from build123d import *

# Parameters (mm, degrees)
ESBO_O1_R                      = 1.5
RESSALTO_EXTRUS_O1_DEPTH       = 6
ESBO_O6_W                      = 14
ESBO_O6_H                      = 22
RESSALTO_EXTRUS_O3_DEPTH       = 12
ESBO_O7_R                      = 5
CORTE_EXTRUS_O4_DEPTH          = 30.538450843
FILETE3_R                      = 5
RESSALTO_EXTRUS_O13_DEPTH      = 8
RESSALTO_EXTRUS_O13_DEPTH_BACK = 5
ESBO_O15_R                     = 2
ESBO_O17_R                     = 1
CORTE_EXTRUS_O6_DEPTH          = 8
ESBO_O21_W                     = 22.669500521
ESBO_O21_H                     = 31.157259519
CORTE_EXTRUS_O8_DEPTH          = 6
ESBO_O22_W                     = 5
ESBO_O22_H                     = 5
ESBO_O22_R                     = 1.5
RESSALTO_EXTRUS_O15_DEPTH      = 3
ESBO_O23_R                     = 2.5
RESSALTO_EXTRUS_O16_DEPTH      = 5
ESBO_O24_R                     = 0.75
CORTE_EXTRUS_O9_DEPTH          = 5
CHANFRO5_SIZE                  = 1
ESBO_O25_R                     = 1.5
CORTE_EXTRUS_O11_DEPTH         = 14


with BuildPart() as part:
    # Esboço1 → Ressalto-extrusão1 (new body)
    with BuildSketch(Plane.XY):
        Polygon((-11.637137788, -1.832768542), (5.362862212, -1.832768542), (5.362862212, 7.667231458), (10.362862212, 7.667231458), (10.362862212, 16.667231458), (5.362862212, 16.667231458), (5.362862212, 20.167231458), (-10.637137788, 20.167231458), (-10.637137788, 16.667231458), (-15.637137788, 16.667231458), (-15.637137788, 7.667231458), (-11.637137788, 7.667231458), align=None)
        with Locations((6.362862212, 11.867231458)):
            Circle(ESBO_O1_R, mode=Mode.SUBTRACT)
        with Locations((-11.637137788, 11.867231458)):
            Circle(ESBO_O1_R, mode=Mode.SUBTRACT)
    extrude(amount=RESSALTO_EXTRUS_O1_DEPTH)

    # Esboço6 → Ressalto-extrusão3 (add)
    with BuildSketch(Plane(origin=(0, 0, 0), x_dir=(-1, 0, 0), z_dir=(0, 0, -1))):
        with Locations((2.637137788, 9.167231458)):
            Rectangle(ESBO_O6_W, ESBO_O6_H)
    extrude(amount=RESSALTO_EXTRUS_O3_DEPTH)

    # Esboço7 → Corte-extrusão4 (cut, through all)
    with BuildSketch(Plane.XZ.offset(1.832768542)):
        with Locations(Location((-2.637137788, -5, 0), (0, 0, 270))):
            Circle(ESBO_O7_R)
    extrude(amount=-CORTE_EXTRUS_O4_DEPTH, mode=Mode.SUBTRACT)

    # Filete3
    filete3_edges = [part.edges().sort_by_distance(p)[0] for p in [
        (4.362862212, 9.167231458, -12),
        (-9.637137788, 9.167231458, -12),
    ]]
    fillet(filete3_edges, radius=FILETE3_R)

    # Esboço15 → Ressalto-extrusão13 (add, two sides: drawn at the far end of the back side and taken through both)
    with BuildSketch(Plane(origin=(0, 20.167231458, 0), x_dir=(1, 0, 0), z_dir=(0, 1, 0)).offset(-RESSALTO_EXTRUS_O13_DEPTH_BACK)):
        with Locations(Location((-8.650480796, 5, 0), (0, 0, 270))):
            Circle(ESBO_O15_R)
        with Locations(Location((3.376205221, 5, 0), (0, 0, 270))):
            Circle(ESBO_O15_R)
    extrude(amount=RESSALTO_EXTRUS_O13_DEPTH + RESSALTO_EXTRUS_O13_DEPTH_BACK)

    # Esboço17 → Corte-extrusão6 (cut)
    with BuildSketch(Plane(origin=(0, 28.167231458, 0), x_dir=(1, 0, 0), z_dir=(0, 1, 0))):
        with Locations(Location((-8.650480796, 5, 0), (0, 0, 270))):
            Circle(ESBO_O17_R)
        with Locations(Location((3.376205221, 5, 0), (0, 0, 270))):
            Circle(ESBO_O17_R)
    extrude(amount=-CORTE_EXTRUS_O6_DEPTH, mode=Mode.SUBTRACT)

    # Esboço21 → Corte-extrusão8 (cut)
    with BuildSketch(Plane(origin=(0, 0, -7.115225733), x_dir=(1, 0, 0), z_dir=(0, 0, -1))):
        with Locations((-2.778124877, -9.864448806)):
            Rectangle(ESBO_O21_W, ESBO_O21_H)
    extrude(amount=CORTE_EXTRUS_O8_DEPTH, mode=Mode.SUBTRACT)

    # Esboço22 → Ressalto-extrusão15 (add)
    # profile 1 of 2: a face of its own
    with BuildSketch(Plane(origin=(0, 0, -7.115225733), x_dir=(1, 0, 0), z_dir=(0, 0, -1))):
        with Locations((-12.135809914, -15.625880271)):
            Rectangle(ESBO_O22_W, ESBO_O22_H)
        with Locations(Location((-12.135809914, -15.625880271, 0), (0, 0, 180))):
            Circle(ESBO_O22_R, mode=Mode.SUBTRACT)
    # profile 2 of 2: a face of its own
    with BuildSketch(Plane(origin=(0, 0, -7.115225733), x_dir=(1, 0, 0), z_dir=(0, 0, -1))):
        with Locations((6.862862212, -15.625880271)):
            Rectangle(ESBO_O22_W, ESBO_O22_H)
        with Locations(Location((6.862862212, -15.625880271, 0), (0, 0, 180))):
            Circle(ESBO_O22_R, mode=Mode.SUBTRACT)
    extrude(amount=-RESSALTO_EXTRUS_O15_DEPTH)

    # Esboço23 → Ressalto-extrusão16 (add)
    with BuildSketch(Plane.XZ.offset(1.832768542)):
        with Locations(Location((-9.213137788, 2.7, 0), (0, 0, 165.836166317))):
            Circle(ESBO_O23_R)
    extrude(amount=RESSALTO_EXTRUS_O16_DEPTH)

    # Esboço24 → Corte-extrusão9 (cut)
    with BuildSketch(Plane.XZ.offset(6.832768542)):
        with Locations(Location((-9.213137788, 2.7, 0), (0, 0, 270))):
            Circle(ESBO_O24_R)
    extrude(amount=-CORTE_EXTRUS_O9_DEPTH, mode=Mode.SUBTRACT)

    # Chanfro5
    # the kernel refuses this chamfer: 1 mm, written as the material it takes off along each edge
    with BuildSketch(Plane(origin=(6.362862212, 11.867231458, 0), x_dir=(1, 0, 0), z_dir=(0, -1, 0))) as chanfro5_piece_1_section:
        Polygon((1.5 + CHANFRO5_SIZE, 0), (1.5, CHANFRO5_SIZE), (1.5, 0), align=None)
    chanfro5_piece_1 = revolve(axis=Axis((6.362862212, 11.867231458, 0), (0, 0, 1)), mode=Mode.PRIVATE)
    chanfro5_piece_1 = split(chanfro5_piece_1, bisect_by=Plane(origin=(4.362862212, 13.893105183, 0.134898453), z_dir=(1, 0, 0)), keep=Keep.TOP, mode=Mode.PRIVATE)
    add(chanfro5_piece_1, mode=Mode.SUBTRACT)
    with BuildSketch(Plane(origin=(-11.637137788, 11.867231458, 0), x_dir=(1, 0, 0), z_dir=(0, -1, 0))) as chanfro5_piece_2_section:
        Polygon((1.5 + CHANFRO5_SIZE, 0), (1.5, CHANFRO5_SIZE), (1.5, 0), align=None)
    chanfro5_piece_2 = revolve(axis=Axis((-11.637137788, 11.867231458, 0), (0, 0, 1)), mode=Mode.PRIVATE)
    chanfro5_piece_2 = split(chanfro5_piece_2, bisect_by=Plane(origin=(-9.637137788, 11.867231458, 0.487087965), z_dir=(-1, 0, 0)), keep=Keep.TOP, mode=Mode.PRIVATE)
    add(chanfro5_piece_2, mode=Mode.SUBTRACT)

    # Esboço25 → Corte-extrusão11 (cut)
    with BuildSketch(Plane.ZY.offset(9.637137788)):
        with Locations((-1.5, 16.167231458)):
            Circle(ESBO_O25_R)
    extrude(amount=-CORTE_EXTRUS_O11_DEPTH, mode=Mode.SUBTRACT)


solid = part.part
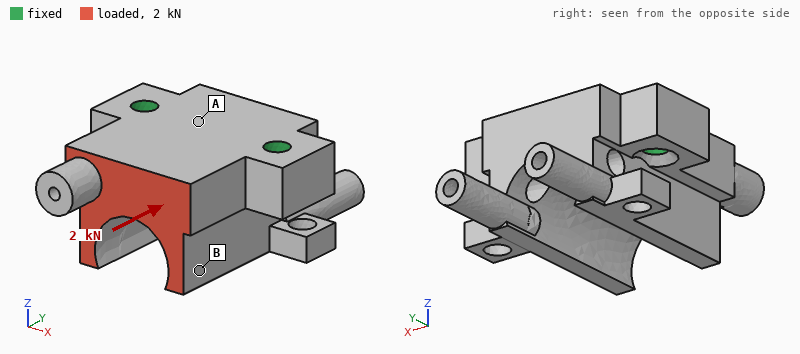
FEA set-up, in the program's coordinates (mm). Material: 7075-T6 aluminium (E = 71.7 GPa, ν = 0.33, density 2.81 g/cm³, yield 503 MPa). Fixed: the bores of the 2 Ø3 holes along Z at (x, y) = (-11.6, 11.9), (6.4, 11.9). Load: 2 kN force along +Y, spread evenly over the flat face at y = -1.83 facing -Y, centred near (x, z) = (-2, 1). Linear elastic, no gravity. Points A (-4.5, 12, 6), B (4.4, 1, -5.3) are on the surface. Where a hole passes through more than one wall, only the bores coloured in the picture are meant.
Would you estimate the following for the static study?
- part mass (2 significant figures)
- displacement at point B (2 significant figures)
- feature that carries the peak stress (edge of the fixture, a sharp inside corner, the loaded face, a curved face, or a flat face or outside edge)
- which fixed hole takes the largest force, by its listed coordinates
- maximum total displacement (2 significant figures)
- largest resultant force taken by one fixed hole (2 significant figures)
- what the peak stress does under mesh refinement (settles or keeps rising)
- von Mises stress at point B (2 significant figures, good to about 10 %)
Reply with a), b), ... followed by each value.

a) 11 g
b) 14 µm
c) edge of the fixture
d) (6.4, 11.9)
e) 17 µm
f) 1.1 kN
g) keeps rising
h) 16 MPa
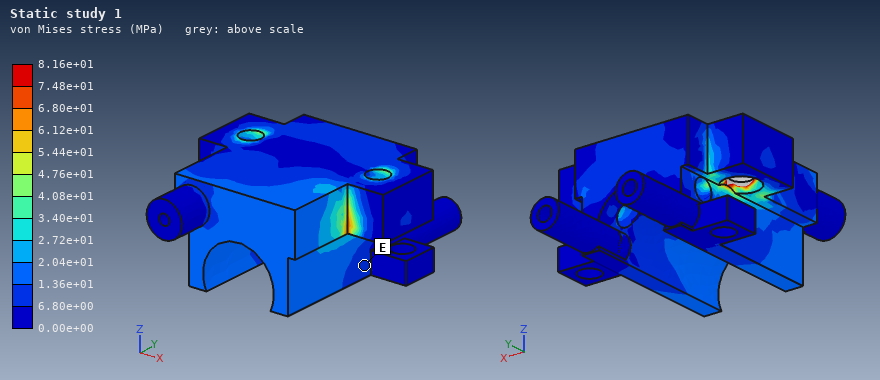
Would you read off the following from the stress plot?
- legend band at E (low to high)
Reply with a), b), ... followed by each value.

a) 6.80e+00 to 1.36e+01 MPa
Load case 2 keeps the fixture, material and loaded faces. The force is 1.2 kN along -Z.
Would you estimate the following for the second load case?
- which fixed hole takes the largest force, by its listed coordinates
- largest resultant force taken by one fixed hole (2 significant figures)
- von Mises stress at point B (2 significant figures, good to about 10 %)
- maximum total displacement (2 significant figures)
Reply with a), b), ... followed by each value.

a) (6.4, 11.9)
b) 680 N
c) 19 MPa
d) 64 µm
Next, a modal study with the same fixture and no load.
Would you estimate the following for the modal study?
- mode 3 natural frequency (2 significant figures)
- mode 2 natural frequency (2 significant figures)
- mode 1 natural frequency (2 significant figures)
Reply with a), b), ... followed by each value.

a) 16 kHz
b) 16 kHz
c) 14 kHz
